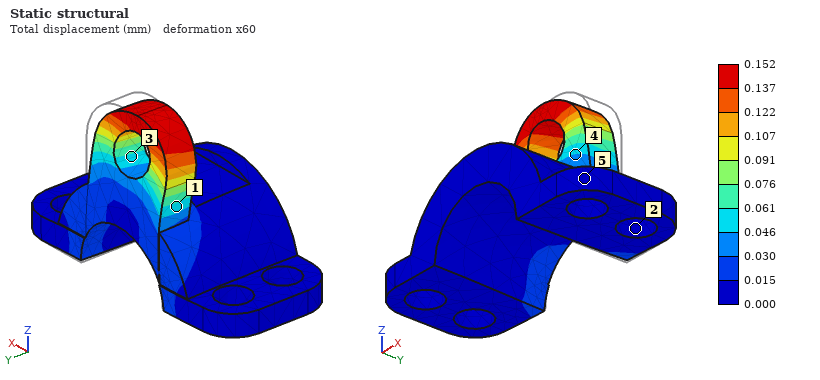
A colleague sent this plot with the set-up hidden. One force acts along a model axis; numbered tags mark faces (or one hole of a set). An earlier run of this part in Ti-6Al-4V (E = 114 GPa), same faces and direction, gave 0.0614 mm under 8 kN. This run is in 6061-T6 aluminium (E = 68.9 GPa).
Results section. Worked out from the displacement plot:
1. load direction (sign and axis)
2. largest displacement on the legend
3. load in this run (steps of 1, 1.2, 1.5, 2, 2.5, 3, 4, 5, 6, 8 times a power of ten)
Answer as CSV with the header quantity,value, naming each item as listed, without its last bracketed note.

quantity,value
load direction,-X
largest displacement on the legend,0.152 mm
load in this run,12 kN
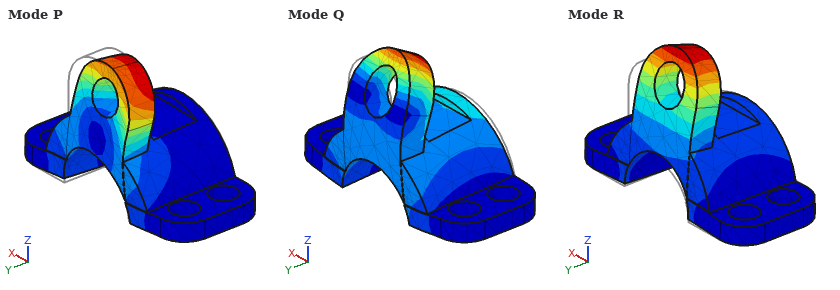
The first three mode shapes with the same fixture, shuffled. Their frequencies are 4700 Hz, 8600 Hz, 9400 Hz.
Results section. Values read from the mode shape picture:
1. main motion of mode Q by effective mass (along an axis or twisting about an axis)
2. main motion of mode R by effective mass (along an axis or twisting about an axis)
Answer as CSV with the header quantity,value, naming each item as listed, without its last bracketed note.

quantity,value
main motion of mode Q by effective mass,along Y
main motion of mode R by effective mass,along Y
